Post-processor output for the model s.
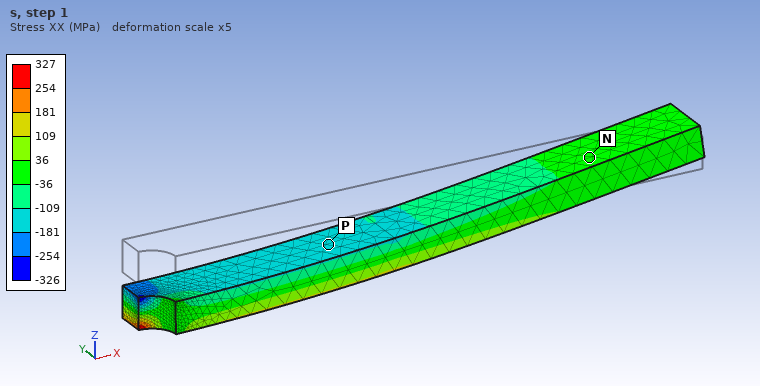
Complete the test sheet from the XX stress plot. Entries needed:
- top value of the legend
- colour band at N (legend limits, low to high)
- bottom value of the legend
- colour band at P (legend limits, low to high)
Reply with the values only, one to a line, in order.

327 MPa
-36 to 36 MPa
-326 MPa
-181 to -109 MPa
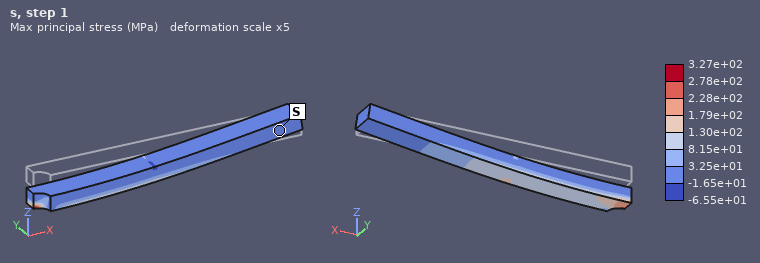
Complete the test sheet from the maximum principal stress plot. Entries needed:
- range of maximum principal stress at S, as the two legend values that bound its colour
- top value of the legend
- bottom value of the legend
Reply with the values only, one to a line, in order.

-1.65e+01 to 3.25e+01 MPa
3.27e+02 MPa
-6.55e+01 MPa
